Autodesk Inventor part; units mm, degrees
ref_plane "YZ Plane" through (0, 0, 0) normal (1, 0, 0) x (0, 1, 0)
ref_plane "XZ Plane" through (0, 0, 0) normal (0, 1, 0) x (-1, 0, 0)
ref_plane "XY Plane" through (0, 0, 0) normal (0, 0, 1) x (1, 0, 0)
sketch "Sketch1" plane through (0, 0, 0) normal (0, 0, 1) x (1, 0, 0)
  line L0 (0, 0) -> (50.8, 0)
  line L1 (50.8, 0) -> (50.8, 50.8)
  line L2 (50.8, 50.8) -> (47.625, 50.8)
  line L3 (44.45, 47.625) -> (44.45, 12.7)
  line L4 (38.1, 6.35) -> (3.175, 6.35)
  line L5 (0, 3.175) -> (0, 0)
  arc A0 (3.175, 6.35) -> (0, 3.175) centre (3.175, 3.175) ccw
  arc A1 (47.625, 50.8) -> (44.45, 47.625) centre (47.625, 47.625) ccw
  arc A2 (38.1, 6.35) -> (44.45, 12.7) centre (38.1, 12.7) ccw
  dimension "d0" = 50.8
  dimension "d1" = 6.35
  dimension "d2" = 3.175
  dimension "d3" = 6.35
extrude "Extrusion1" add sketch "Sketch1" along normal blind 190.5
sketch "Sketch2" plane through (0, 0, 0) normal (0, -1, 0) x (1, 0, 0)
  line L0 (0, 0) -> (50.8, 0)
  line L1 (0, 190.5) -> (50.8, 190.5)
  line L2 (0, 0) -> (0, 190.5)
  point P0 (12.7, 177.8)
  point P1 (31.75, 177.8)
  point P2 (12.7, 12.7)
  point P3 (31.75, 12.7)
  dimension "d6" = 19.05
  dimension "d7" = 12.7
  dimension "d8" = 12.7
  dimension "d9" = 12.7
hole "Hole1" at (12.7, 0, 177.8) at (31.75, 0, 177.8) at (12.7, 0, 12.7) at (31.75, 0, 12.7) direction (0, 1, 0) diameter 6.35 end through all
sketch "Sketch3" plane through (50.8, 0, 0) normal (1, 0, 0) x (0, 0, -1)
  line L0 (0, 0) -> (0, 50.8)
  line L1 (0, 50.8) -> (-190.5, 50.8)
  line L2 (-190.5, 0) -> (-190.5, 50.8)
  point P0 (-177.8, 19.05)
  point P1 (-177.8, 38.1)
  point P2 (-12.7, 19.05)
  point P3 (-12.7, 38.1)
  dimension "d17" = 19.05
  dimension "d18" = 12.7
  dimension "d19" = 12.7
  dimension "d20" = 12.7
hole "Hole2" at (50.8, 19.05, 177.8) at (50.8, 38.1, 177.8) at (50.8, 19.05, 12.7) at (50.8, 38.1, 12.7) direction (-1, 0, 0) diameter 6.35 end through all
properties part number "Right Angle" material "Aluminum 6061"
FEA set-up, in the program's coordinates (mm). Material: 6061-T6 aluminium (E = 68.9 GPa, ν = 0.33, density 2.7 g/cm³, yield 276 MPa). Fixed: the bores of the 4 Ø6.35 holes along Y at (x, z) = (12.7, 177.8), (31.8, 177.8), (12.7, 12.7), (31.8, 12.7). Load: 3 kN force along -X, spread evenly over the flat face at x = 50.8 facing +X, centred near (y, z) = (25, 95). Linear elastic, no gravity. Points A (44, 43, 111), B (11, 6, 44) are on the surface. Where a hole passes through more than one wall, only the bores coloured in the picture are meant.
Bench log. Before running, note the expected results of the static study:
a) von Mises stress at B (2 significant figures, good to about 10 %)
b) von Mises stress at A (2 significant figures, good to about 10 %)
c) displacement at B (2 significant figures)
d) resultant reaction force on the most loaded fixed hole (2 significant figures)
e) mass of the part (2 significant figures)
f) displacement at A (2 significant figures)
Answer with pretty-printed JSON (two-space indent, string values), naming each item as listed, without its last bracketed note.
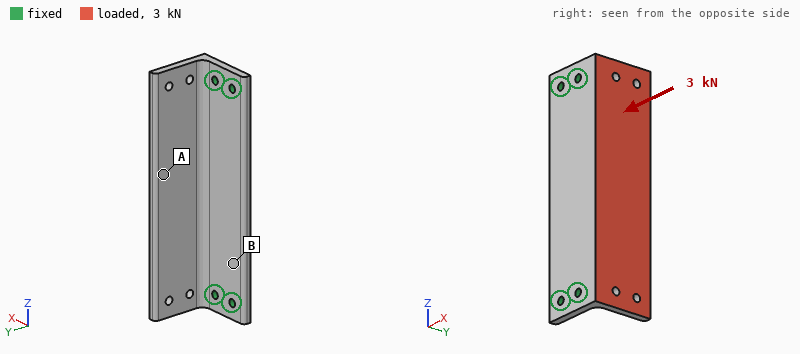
{
  "von Mises stress at B": "31 MPa",
  "von Mises stress at A": "12 MPa",
  "displacement at B": "0.072 mm",
  "resultant reaction force on the most loaded fixed hole": "1.6 kN",
  "mass of the part": "310 g",
  "displacement at A": "0.34 mm"
}
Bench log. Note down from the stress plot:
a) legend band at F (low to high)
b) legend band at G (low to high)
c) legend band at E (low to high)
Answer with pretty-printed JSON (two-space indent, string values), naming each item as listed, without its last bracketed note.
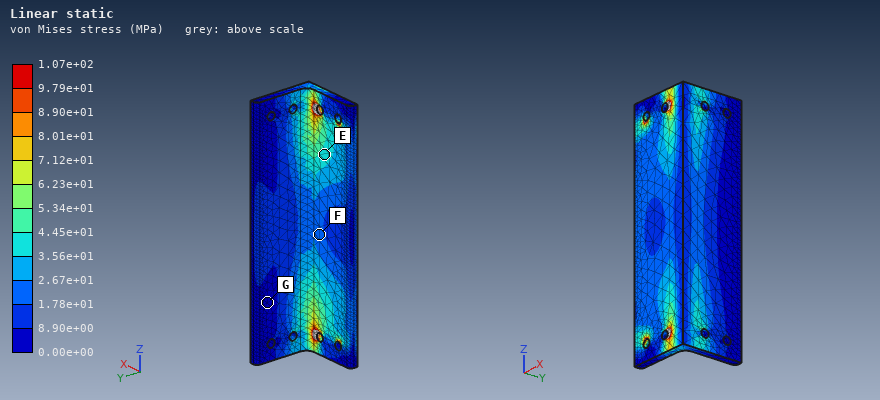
{
  "legend band at F": "1.78e+01 to 2.67e+01 MPa",
  "legend band at G": "0.00e+00 to 8.90e+00 MPa",
  "legend band at E": "3.56e+01 to 4.45e+01 MPa"
}
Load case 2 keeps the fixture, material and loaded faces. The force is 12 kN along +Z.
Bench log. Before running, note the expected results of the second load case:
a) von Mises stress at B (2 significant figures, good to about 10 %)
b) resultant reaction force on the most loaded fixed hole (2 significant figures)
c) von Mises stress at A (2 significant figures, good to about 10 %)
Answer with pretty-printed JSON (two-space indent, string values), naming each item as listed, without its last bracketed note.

{
  "von Mises stress at B": "10 MPa",
  "resultant reaction force on the most loaded fixed hole": "4.8 kN",
  "von Mises stress at A": "7.2 MPa"
}
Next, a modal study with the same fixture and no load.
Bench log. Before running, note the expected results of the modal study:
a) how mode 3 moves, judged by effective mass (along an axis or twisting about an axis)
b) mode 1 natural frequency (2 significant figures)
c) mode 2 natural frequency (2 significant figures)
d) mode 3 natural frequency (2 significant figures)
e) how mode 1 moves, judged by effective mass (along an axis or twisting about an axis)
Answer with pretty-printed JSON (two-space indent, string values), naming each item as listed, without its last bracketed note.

{
  "how mode 3 moves, judged by effective mass": "along Y",
  "mode 1 natural frequency": "1200 Hz",
  "mode 2 natural frequency": "2100 Hz",
  "mode 3 natural frequency": "2300 Hz",
  "how mode 1 moves, judged by effective mass": "along X"
}
